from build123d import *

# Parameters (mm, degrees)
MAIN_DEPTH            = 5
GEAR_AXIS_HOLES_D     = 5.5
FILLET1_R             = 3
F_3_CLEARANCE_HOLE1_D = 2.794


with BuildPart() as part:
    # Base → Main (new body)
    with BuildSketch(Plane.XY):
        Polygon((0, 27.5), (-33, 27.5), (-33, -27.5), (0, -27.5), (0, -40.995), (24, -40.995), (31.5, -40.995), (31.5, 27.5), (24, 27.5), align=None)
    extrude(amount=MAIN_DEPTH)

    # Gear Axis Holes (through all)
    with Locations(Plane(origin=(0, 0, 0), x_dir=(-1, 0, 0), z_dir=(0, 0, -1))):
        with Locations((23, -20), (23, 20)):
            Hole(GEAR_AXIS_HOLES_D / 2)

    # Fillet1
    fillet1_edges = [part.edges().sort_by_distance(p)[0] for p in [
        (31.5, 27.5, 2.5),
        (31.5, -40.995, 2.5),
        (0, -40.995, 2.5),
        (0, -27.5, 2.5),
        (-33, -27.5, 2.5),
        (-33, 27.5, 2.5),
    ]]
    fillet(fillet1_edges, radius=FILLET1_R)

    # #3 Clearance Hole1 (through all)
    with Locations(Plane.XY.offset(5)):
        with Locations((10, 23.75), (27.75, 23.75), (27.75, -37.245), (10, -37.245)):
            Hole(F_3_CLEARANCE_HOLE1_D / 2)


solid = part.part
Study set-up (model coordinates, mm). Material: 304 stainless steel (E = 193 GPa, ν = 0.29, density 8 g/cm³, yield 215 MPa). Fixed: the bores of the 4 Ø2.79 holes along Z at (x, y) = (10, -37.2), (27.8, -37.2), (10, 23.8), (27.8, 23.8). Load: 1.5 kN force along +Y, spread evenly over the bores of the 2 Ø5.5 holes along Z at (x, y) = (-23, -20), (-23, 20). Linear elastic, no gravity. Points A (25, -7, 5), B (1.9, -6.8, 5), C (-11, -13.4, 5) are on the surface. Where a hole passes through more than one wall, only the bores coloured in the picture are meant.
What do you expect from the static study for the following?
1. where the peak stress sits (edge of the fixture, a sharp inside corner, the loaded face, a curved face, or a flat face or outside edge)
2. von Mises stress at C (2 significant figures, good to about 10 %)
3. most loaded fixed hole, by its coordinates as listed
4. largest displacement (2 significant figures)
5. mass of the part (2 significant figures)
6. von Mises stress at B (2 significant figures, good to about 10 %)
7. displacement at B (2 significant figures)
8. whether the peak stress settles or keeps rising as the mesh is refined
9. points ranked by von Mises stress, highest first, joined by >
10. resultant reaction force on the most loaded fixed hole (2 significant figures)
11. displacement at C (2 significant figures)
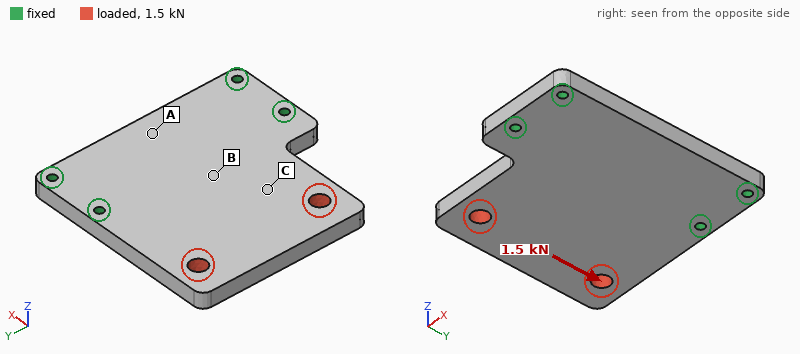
edge of the fixture
13 MPa
(10, 23.8)
6.0 µm
160 g
7.2 MPa
1.3 µm
keeps rising
C > B > A
1.0 kN
2.9 µm
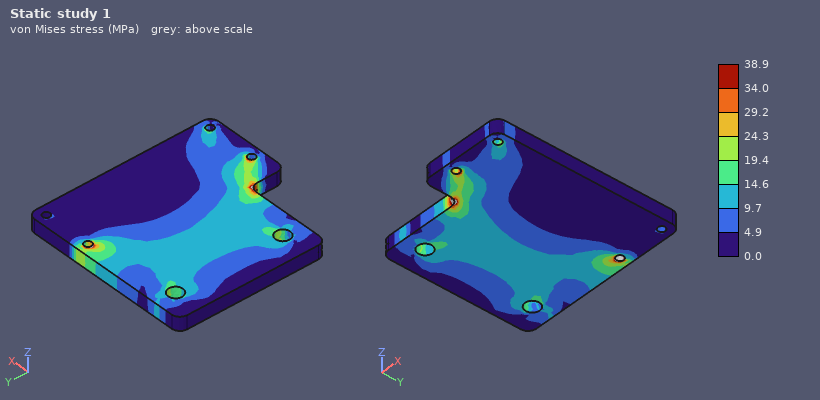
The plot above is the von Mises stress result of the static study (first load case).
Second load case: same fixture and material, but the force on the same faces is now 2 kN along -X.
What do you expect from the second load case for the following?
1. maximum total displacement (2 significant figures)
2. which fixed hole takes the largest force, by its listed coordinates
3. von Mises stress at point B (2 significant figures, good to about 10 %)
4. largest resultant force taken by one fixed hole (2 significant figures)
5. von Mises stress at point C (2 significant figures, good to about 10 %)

3.4 µm
(10, 23.8)
3.7 MPa
930 N
5.7 MPa
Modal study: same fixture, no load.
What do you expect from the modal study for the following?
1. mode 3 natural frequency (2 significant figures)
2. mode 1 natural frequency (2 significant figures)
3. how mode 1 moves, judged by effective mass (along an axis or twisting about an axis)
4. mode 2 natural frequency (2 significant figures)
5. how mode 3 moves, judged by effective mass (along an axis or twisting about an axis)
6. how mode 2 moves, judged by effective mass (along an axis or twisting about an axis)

6300 Hz
1700 Hz
along Z
4200 Hz
along Z
twisting about X
